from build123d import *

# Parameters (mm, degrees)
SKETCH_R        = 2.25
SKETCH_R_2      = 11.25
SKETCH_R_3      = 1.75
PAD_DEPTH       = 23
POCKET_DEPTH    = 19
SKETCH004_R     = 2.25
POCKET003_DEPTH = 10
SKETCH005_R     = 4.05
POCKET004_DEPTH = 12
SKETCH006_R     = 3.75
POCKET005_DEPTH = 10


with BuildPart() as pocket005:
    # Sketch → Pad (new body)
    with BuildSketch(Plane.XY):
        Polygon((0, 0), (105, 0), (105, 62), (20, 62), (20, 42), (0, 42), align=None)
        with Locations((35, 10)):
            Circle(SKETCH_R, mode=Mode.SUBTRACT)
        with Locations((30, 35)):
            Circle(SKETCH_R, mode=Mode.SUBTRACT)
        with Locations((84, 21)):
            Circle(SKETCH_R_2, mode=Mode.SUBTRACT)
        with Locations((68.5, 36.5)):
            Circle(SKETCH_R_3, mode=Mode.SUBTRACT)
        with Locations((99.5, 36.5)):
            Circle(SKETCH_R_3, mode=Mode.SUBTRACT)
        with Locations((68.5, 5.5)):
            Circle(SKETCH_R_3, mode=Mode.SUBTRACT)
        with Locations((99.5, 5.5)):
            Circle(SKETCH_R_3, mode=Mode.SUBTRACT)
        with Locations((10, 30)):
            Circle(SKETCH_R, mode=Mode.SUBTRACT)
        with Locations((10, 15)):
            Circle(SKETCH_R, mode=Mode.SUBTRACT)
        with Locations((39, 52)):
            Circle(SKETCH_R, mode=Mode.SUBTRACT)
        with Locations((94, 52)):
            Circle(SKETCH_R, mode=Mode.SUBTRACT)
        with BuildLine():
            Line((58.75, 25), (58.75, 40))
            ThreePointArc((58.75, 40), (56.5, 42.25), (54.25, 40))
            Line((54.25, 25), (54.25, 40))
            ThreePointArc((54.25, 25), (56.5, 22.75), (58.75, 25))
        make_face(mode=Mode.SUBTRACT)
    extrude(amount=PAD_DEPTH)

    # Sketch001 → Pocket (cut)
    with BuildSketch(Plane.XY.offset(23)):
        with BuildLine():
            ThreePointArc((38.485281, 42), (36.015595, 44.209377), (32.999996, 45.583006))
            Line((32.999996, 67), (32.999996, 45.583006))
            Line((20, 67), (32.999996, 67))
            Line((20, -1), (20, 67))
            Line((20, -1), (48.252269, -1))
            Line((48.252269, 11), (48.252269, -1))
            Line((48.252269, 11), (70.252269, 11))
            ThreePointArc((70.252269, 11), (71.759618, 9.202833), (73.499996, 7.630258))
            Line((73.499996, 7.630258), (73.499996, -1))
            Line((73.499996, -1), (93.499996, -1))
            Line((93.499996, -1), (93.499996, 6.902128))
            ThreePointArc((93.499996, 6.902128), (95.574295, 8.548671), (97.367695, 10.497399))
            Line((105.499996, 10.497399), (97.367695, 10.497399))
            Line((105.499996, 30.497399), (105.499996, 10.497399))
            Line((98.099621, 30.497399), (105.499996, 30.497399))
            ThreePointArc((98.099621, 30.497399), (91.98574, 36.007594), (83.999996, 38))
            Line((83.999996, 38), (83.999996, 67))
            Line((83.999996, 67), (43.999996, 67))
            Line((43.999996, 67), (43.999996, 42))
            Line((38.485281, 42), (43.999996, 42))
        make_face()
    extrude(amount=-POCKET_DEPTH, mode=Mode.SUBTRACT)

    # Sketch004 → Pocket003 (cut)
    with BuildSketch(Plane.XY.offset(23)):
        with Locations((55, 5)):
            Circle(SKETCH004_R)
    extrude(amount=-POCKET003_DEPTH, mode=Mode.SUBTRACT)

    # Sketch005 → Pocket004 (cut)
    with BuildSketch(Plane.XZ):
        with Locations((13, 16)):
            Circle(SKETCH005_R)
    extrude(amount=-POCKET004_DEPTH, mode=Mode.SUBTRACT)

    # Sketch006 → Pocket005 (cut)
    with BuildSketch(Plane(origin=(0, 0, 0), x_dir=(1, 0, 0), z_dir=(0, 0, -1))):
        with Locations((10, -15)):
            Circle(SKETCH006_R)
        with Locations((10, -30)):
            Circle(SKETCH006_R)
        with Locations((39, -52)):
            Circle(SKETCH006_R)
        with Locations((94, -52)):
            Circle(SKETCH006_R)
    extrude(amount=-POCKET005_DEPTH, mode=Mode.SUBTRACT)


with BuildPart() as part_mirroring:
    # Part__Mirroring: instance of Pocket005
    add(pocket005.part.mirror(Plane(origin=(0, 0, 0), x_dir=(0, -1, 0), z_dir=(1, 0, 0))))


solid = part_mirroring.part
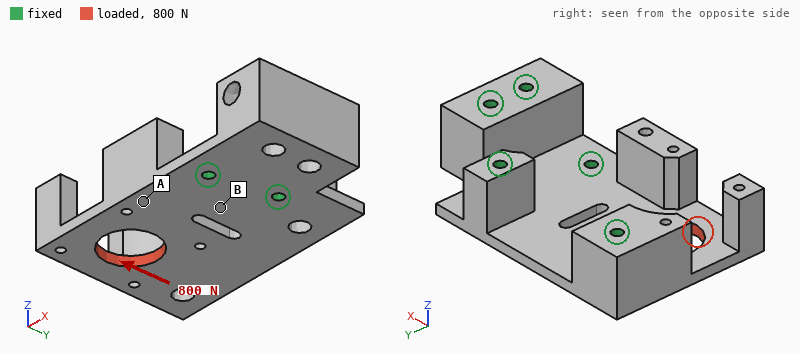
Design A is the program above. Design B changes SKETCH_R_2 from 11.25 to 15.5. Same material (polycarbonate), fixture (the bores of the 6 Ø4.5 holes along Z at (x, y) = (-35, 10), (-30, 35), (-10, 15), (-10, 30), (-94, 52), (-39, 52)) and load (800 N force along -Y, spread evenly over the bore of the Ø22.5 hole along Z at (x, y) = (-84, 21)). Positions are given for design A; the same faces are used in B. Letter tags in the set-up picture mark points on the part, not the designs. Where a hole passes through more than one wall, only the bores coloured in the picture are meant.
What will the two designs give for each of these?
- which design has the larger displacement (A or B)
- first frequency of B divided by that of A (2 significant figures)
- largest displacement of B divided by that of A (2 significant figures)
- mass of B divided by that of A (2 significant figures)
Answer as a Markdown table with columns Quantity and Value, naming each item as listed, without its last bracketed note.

| Quantity | Value |
|---|---|
| which design has the larger displacement | B |
| first frequency of B divided by that of A | 0.86 |
| largest displacement of B divided by that of A | 1.2 |
| mass of B divided by that of A | 0.97 |
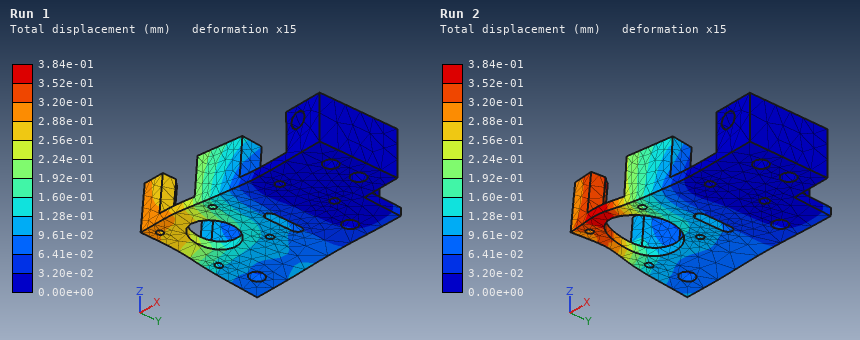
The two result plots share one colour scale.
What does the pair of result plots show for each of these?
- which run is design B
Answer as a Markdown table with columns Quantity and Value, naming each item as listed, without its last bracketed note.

| Quantity | Value |
|---|---|
| which run is design B | Run 2 |
